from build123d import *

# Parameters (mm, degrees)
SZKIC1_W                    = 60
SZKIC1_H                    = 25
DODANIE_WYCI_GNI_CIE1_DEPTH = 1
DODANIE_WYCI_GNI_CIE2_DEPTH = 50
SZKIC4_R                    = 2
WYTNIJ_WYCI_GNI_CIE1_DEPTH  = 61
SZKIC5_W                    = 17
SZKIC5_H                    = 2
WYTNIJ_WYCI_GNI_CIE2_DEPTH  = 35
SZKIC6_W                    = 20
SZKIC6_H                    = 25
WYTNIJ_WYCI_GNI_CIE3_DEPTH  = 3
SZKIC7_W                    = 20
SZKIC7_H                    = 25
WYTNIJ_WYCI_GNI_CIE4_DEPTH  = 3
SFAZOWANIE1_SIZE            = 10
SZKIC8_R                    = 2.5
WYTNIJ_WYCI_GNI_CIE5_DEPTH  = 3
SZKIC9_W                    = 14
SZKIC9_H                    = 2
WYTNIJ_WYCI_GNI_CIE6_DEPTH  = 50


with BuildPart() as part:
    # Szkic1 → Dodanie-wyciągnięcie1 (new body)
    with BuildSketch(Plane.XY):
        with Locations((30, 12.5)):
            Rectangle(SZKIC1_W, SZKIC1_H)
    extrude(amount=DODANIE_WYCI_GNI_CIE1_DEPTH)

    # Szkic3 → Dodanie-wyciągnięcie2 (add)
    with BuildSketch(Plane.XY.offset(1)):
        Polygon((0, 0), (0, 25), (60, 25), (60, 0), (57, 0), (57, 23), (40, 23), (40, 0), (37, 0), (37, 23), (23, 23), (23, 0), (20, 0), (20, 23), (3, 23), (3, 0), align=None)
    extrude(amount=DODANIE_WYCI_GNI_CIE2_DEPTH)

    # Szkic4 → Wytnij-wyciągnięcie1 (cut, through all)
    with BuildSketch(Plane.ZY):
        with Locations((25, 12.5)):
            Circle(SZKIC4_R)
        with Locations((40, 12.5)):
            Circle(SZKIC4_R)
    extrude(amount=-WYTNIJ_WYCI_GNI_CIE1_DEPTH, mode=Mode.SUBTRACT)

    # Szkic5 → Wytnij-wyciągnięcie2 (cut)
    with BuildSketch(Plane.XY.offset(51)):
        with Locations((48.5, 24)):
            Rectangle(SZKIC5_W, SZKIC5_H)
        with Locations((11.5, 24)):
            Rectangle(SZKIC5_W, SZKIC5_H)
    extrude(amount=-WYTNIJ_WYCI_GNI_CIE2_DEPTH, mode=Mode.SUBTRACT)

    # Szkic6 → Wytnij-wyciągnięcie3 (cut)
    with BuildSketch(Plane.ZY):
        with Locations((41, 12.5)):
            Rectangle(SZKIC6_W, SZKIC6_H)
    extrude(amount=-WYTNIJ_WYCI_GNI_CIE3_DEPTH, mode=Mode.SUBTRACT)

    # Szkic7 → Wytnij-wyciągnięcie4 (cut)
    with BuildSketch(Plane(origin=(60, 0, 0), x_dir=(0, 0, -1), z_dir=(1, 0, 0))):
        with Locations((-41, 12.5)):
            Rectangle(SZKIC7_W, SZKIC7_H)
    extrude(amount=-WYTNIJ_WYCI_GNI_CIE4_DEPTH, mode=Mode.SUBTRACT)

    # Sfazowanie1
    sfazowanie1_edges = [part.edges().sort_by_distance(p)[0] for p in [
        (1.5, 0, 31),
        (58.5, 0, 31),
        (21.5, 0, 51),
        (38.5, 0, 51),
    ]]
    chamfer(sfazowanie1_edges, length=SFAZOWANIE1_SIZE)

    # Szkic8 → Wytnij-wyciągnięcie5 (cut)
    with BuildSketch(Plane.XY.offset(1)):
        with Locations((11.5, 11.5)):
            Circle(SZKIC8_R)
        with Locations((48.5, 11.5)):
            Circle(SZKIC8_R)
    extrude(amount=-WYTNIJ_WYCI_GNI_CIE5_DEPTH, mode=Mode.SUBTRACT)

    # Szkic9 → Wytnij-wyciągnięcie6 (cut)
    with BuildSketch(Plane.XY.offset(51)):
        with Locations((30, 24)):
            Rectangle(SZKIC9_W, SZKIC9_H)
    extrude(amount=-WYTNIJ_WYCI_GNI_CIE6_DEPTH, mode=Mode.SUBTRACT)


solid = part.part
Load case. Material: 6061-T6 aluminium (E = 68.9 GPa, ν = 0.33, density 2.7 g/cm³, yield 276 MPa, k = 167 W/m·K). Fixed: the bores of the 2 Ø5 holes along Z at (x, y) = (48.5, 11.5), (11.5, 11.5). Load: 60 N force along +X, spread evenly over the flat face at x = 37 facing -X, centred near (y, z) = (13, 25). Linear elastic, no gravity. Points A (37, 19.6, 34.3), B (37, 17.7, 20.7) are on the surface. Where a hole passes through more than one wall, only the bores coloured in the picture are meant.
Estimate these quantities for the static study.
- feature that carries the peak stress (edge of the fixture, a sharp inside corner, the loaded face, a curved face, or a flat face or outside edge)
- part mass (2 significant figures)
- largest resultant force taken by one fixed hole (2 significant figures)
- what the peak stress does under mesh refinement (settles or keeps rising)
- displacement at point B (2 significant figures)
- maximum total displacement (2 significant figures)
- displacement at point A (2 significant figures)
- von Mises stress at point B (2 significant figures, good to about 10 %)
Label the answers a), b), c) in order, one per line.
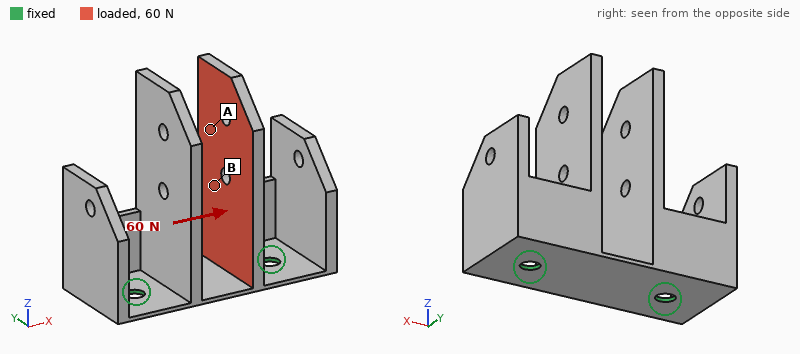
a) edge of the fixture
b) 37 g
c) 48 N
d) keeps rising
e) 0.22 mm
f) 0.62 mm
g) 0.38 mm
h) 20 MPa
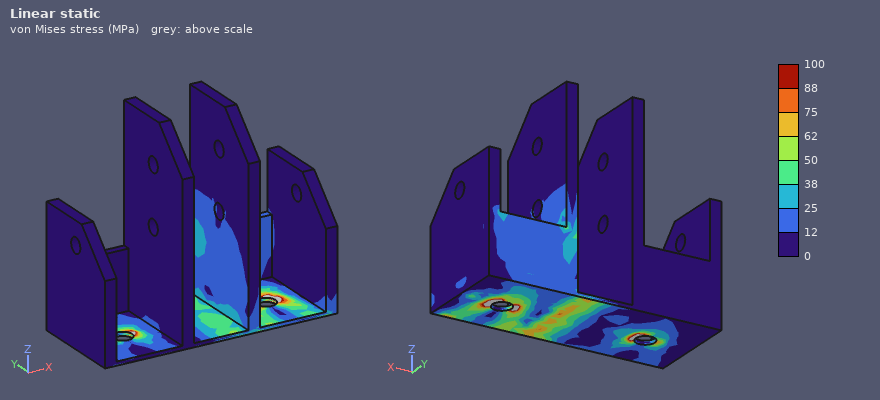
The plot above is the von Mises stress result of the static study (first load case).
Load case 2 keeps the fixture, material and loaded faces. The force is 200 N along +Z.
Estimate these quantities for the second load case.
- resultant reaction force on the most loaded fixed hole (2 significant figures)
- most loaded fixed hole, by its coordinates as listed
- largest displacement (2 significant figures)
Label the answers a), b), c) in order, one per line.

a) 150 N
b) (48.5, 11.5)
c) 0.57 mm
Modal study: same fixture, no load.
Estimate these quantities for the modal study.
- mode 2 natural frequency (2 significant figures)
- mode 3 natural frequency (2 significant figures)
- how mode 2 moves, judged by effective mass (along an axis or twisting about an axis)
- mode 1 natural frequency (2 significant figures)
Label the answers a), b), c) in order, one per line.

a) 530 Hz
b) 740 Hz
c) along Y
d) 470 Hz
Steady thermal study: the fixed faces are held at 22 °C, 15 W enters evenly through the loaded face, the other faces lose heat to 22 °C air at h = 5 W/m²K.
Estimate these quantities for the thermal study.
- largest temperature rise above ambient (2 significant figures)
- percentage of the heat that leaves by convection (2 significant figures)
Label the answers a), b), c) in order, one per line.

a) 47 K
b) 4.8 %
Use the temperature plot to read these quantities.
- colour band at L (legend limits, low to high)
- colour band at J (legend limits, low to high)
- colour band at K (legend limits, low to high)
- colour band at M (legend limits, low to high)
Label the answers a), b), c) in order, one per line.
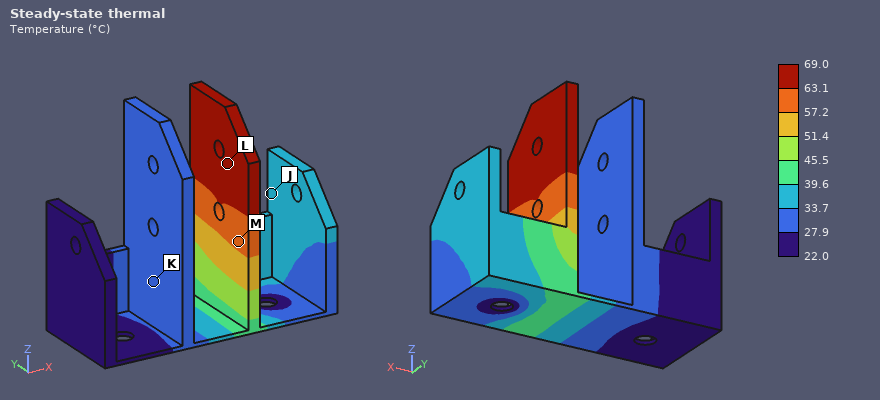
a) 63.1 to 69.0 °C
b) 33.7 to 39.6 °C
c) 27.9 to 33.7 °C
d) 57.2 to 63.1 °C
